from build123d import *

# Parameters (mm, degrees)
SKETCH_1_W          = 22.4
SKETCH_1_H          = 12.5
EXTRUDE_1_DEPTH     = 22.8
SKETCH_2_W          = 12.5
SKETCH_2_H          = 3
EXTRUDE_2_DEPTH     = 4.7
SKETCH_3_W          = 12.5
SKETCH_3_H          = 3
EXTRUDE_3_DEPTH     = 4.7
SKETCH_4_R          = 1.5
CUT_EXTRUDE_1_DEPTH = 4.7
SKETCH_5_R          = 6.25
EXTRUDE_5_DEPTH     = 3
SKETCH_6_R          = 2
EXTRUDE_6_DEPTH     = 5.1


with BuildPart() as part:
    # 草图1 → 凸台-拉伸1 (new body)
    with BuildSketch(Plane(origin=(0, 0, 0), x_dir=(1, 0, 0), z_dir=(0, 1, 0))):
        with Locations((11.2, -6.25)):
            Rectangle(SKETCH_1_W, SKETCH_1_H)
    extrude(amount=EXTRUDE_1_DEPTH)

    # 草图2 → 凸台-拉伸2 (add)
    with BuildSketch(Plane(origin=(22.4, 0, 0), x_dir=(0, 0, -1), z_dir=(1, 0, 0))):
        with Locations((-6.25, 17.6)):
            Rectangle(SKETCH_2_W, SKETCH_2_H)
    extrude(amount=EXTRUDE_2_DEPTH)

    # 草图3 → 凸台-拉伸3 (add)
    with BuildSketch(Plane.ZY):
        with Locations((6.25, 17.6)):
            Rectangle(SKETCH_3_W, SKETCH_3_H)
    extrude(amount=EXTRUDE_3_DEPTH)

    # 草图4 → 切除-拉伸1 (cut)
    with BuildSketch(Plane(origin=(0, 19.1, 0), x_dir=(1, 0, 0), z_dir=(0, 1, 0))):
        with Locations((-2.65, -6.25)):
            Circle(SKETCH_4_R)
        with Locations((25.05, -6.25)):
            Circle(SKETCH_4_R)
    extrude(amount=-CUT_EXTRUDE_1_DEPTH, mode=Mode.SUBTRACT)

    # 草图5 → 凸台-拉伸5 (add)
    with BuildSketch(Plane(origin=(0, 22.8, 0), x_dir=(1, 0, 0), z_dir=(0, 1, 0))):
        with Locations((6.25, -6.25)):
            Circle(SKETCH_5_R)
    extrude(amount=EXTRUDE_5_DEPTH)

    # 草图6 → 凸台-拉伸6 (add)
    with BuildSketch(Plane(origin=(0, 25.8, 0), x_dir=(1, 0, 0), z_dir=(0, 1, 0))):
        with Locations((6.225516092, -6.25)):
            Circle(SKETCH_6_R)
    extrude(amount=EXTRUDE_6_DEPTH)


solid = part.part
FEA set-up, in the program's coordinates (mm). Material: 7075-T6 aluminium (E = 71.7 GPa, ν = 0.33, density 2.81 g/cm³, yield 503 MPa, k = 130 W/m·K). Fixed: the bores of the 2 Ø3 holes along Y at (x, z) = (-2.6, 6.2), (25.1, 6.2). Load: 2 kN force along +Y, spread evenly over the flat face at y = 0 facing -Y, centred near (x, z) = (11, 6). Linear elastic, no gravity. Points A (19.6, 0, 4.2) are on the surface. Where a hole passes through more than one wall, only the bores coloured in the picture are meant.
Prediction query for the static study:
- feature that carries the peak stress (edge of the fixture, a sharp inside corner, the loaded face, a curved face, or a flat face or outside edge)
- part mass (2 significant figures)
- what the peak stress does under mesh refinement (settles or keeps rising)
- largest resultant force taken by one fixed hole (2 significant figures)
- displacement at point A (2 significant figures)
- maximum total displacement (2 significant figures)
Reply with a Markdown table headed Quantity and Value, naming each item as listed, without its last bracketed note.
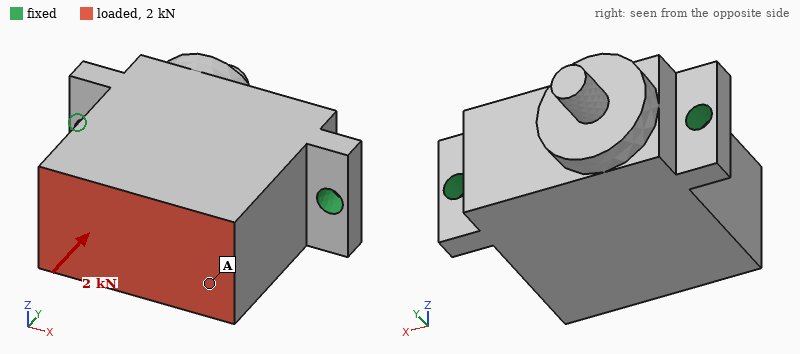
| Quantity | Value |
|---|---|
| feature that carries the peak stress | edge of the fixture |
| part mass | 20 g |
| what the peak stress does under mesh refinement | keeps rising |
| largest resultant force taken by one fixed hole | 1.0 kN |
| displacement at point A | 8.7 µm |
| maximum total displacement | 8.8 µm |
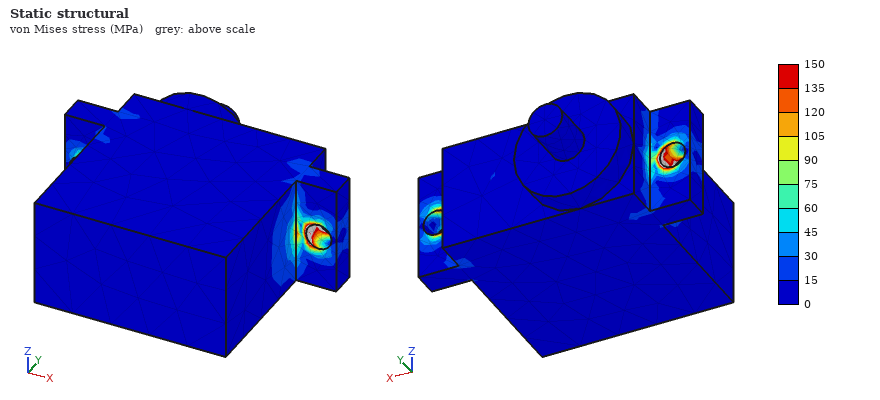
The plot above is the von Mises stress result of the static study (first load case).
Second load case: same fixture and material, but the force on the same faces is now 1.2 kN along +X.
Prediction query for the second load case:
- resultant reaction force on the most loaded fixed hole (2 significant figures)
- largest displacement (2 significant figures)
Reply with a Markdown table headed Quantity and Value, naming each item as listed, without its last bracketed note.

| Quantity | Value |
|---|---|
| resultant reaction force on the most loaded fixed hole | 1.1 kN |
| largest displacement | 16 µm |
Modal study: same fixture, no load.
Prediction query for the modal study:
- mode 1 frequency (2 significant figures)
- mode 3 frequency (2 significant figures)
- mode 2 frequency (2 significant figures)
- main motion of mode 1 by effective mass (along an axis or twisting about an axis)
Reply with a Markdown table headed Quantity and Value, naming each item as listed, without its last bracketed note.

| Quantity | Value |
|---|---|
| mode 1 frequency | 5300 Hz |
| mode 3 frequency | 19 kHz |
| mode 2 frequency | 19 kHz |
| main motion of mode 1 by effective mass | along Z |
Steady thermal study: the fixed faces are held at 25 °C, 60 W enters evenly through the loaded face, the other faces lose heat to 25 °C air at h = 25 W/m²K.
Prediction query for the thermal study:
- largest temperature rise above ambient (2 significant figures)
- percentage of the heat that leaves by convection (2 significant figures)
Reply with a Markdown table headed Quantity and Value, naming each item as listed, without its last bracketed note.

| Quantity | Value |
|---|---|
| largest temperature rise above ambient | 56 K |
| percentage of the heat that leaves by convection | 3.1 % |
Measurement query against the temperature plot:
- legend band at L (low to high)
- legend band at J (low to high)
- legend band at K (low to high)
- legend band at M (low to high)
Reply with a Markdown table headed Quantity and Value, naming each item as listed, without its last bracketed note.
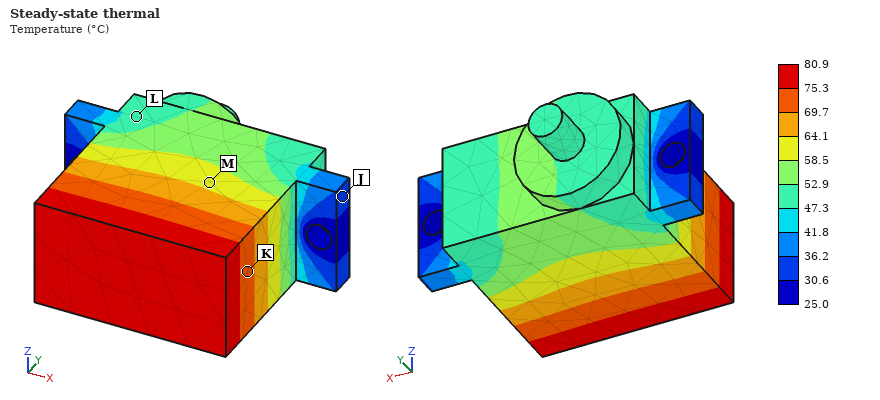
| Quantity | Value |
|---|---|
| legend band at L | 47.3 to 52.9 °C |
| legend band at J | 30.6 to 36.2 °C |
| legend band at K | 69.7 to 75.3 °C |
| legend band at M | 58.5 to 64.1 °C |
